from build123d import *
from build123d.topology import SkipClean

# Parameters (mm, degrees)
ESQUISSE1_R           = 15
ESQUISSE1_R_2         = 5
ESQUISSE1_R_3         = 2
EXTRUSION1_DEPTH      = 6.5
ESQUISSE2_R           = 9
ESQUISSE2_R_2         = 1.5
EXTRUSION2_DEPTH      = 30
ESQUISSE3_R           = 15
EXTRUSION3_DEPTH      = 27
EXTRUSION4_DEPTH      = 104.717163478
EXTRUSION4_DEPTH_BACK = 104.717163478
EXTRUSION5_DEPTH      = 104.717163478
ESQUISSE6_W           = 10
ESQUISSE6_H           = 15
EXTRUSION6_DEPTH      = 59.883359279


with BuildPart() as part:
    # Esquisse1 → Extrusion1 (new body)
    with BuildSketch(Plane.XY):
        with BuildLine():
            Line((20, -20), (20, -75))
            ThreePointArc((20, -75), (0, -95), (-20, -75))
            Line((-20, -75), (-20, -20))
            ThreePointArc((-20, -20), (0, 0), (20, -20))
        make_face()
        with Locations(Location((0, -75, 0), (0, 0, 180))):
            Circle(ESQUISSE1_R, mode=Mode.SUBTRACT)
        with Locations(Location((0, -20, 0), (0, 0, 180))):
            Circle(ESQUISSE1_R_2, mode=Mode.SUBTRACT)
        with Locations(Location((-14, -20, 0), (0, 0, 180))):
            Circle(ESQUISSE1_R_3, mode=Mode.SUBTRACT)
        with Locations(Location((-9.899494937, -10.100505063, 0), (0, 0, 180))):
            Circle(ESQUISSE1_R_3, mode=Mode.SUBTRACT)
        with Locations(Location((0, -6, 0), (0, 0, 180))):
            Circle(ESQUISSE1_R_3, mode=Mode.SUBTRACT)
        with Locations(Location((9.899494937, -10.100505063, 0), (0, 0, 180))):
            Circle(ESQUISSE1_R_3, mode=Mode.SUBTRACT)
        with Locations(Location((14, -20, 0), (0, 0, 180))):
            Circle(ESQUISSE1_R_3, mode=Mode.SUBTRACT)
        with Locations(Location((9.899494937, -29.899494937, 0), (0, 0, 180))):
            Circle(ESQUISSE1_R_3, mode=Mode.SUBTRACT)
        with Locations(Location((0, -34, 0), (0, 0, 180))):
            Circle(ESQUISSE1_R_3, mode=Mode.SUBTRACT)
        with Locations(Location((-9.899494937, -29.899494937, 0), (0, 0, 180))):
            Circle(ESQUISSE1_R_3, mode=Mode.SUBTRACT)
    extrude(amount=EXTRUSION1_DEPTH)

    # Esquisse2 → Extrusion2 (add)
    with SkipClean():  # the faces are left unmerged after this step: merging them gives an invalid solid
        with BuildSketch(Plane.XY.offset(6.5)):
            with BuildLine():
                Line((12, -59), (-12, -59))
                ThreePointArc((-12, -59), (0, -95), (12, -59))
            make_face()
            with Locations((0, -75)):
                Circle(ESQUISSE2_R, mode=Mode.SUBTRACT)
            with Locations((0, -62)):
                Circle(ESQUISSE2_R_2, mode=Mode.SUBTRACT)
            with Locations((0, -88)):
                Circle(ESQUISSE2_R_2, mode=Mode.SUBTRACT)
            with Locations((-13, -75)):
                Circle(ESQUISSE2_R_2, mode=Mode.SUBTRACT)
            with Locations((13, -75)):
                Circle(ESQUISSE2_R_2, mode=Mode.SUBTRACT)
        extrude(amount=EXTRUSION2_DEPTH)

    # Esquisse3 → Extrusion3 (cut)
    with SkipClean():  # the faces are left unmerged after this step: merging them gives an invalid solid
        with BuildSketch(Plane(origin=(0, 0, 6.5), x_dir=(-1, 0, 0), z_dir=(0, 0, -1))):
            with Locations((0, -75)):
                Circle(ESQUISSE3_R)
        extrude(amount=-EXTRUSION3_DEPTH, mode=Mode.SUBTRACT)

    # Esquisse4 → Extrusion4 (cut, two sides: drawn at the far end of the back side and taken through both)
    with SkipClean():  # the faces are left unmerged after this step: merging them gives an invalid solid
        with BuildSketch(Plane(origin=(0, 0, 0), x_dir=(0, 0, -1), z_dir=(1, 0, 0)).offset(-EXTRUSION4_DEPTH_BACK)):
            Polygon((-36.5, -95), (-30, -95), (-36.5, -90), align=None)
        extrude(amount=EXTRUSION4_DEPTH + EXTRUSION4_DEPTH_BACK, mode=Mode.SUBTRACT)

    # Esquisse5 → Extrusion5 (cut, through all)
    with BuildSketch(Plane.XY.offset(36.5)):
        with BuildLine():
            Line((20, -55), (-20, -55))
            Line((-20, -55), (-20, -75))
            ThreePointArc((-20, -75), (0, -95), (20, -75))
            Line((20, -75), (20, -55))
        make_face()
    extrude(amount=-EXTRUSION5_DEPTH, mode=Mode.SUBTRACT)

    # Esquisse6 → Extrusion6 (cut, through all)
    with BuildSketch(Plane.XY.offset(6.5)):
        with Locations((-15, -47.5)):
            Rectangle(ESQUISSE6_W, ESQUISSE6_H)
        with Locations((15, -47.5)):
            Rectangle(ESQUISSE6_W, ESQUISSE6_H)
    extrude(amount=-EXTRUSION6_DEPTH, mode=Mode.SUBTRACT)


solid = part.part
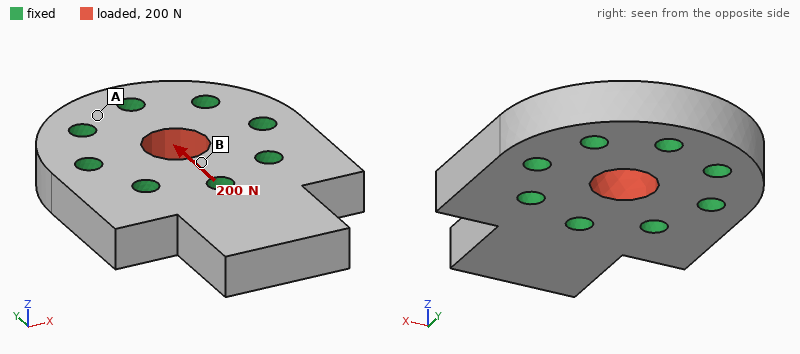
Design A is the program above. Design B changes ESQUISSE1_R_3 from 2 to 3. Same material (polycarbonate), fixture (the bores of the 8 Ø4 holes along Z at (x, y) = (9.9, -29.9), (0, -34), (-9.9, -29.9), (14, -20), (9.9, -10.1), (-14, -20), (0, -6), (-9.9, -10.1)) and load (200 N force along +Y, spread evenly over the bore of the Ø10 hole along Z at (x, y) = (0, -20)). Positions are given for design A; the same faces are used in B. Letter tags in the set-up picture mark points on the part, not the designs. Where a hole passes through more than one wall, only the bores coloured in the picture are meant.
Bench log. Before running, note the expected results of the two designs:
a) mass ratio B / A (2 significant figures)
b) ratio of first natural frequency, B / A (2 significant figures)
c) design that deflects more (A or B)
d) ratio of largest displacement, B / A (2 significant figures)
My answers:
0.92
1.1
A
0.87
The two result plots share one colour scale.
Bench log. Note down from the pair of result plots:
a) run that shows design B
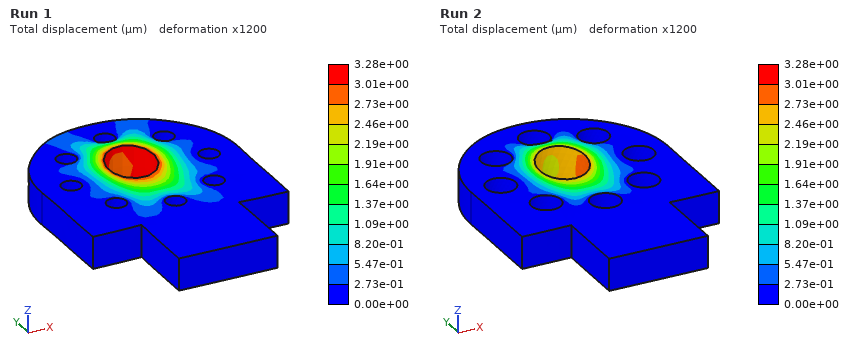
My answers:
Run 2
